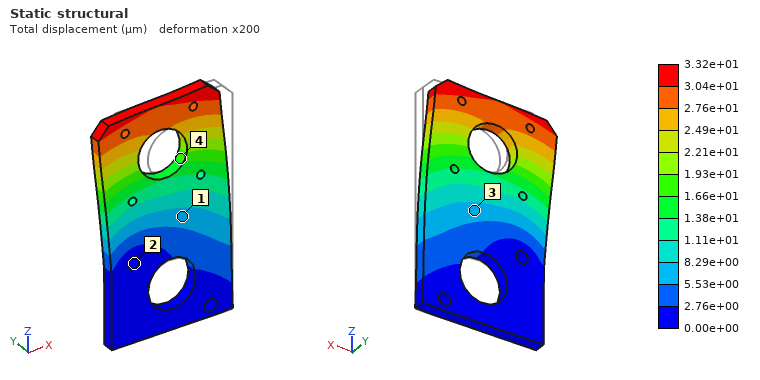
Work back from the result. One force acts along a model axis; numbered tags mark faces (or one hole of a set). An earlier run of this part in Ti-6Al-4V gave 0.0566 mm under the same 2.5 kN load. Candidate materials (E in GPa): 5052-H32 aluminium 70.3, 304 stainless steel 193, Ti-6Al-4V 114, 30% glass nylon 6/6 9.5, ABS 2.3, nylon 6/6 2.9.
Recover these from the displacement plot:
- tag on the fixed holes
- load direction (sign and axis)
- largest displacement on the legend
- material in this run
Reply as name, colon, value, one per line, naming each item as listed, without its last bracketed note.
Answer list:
tag on the fixed holes: 2
load direction: -X
largest displacement on the legend: 3.32e+01 µm
material in this run: 304 stainless steel
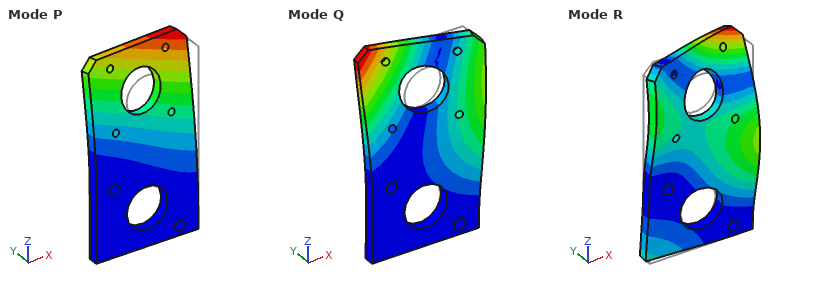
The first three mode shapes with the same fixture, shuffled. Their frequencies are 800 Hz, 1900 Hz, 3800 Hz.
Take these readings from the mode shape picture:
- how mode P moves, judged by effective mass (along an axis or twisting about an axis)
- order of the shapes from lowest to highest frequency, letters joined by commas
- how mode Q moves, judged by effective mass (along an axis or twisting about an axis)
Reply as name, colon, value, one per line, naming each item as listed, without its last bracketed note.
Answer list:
how mode P moves, judged by effective mass: along Y
order of the shapes from lowest to highest frequency, letters joined by commas: P, Q, R
how mode Q moves, judged by effective mass: twisting about Z
